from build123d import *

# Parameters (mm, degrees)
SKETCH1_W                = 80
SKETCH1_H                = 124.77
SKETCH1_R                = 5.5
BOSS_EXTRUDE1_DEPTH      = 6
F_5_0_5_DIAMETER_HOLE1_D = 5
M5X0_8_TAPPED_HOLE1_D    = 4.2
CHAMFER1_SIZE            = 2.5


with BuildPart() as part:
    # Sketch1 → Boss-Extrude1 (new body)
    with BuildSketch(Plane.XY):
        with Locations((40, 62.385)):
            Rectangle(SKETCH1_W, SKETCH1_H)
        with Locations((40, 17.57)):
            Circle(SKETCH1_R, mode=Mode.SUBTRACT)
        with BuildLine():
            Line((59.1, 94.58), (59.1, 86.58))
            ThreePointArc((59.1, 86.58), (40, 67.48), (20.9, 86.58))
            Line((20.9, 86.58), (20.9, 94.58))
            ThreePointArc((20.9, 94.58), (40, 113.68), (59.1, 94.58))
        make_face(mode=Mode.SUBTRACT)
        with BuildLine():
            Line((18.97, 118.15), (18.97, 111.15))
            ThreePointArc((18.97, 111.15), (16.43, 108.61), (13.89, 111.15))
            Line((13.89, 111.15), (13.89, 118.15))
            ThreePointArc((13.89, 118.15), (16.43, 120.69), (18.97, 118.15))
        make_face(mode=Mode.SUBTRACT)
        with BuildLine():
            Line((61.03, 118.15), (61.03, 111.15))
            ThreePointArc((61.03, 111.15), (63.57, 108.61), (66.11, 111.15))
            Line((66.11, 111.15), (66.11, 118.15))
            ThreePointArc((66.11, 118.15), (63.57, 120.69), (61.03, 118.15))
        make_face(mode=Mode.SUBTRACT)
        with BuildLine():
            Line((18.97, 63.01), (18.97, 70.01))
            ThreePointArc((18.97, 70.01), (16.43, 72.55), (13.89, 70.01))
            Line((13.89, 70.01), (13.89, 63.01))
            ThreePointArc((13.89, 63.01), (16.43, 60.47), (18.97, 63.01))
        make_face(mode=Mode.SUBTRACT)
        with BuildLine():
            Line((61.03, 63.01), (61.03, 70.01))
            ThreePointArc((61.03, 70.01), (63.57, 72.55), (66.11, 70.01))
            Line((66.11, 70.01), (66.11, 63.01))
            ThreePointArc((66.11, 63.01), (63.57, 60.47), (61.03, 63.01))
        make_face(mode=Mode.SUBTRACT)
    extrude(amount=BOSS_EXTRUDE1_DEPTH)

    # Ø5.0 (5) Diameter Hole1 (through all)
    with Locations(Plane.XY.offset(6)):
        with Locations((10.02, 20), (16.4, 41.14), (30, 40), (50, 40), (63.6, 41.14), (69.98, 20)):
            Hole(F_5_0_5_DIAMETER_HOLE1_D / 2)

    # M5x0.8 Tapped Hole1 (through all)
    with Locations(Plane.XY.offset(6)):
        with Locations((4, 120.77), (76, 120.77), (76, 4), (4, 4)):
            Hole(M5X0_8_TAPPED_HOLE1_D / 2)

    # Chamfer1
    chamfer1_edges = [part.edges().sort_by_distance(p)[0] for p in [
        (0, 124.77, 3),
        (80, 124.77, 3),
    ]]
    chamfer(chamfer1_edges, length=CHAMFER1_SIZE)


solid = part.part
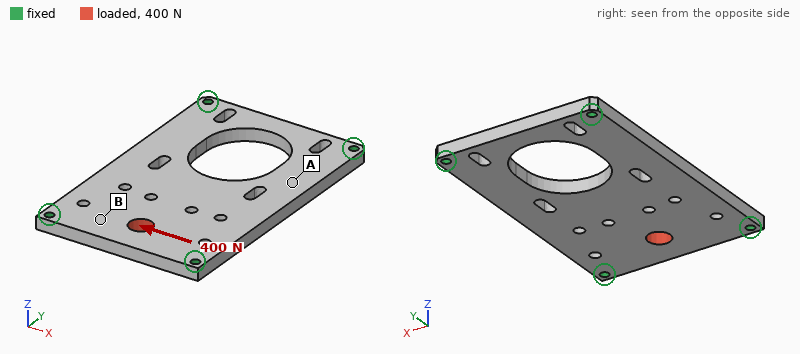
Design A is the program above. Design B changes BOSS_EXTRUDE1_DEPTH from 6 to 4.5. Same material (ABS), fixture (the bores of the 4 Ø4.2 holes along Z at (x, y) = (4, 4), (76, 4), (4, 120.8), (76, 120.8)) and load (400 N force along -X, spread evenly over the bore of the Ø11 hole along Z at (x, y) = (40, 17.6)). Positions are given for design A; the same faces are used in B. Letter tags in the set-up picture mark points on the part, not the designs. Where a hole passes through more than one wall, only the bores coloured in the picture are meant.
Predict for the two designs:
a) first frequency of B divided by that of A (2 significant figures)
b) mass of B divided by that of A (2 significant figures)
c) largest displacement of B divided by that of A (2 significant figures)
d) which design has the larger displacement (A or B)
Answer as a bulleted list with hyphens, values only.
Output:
- 0.77
- 0.75
- 1.3
- B
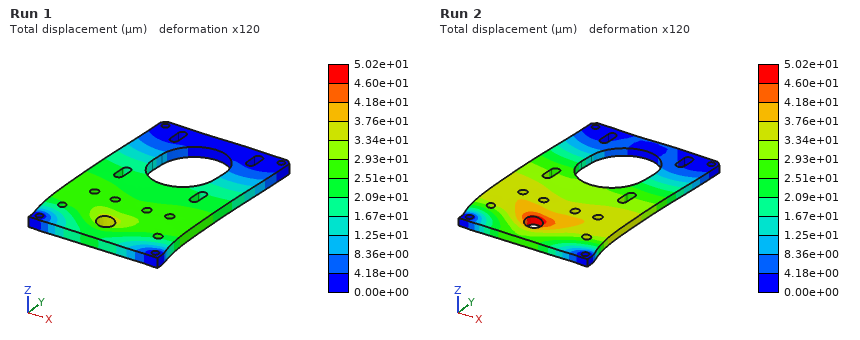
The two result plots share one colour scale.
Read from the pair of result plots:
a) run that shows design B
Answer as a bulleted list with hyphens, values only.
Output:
- Run 2
